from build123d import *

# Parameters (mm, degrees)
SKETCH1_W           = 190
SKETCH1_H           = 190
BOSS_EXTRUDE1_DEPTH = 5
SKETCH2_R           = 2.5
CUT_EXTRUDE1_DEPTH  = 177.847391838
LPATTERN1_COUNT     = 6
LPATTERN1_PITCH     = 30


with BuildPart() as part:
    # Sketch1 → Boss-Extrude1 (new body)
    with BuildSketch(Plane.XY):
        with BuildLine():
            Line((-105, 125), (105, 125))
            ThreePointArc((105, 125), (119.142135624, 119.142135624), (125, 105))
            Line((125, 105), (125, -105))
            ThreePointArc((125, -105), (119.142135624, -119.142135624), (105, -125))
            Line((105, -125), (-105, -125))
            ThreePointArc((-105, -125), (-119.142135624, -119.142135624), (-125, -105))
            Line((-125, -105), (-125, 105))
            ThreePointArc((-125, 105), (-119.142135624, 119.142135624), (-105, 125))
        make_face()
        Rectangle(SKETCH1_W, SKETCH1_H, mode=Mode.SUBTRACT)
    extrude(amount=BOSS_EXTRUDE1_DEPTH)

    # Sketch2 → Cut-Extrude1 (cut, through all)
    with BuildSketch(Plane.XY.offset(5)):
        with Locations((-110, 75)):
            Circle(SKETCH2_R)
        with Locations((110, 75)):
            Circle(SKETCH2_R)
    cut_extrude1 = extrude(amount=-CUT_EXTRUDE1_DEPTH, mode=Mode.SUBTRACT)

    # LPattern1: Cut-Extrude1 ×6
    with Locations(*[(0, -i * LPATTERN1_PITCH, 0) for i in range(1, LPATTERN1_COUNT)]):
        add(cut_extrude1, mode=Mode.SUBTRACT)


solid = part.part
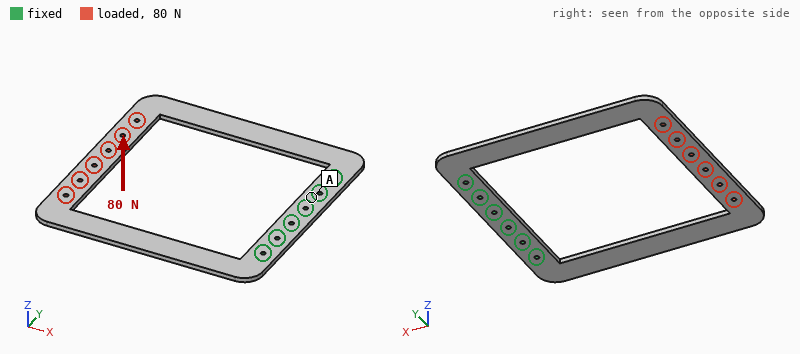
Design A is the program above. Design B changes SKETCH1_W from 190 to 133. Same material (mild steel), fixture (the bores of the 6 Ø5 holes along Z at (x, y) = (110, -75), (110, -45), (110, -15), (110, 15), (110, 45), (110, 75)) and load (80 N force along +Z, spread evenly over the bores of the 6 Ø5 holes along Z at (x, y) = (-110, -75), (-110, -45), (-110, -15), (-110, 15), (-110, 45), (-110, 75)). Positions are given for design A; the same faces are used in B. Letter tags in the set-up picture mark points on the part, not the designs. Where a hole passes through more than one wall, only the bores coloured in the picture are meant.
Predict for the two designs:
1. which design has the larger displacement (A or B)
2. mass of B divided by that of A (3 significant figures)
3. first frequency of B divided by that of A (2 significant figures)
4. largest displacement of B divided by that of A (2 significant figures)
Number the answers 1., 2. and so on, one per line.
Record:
1. A
2. 1.42
3. 1.0
4. 0.71
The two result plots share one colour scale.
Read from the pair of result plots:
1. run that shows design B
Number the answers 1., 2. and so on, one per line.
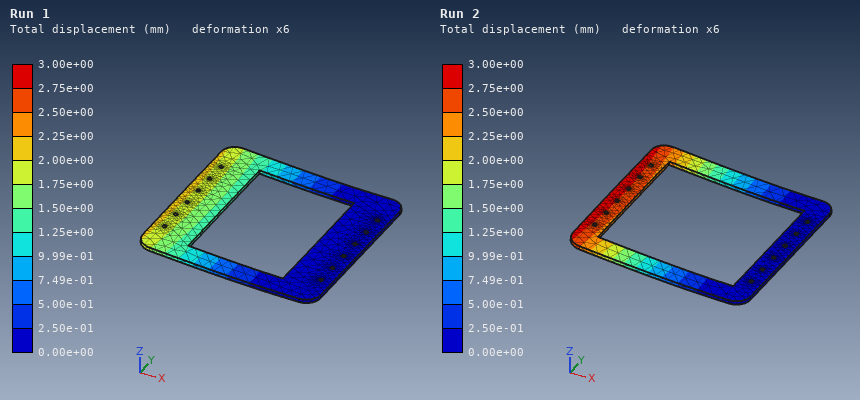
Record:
1. Run 1
